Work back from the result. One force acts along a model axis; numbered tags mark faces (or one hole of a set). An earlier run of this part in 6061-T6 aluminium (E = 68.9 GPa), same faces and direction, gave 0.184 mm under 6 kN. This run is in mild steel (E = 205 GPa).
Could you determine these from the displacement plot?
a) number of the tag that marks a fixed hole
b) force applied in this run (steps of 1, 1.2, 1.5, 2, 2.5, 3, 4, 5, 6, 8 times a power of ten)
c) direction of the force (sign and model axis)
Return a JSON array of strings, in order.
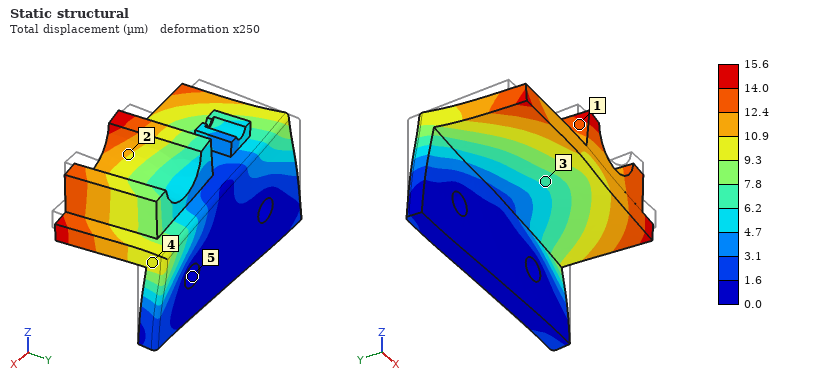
["5", "1.5 kN", "+X"]
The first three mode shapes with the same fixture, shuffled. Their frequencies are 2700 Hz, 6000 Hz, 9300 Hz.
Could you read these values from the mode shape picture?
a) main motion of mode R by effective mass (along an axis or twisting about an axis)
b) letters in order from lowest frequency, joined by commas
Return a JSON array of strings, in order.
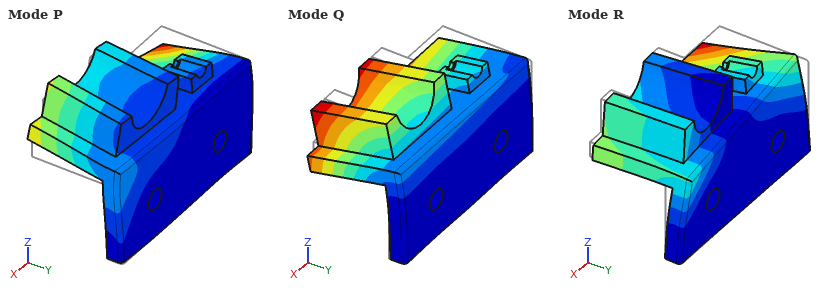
["along X", "Q, R, P"]
